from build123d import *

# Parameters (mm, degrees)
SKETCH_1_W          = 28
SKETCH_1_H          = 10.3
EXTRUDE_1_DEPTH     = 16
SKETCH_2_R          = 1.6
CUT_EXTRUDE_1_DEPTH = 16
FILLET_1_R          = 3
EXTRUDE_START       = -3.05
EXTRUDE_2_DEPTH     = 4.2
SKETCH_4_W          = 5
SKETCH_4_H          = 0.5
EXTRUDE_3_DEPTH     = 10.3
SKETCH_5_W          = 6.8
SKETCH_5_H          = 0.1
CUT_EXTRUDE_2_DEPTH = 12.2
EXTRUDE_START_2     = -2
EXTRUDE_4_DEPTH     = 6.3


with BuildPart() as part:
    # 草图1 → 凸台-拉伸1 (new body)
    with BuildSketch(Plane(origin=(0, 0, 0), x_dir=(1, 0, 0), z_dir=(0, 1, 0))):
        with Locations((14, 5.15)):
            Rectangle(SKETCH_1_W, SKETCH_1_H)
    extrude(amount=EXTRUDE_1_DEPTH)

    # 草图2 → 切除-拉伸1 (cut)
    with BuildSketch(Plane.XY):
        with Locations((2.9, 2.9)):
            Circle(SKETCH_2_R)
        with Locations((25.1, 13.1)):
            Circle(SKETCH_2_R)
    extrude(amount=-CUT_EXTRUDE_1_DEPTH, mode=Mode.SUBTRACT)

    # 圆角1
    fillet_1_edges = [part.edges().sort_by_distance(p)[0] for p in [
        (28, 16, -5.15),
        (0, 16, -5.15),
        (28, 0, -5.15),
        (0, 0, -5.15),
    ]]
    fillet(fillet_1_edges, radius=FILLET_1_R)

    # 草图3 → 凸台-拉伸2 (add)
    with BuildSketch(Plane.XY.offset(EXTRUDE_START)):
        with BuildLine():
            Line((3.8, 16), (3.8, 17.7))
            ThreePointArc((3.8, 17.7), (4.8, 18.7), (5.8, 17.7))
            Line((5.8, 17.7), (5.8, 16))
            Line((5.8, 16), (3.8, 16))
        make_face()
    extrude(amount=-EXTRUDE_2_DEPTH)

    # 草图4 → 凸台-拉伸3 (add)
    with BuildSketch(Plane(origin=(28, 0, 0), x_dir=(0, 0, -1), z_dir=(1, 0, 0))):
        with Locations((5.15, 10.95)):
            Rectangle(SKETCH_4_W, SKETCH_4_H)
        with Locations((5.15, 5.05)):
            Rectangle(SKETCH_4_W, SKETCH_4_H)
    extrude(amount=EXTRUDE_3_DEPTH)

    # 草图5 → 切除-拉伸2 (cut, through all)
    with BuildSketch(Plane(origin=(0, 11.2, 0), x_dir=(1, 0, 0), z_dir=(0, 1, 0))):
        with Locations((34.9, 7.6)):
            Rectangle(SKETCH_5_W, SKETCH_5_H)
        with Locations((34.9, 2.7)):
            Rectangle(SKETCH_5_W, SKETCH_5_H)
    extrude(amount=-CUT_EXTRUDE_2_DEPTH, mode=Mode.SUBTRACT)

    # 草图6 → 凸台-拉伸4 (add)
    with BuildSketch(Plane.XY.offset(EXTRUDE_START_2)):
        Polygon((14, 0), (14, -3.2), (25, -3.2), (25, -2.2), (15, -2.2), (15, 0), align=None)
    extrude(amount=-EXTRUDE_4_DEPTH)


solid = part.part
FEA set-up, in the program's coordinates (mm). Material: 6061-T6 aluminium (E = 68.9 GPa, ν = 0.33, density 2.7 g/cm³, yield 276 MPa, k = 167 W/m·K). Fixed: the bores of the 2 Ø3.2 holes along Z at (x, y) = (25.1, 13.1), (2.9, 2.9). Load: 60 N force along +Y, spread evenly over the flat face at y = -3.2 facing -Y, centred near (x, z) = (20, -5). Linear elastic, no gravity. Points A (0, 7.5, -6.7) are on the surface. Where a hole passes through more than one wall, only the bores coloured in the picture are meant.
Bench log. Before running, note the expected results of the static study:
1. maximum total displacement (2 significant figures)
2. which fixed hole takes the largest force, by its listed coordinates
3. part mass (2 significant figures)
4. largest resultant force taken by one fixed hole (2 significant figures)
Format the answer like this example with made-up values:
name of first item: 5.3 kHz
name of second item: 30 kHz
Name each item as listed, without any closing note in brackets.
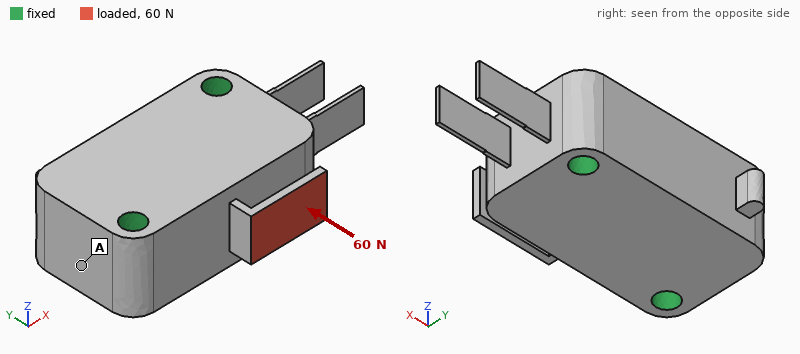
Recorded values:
maximum total displacement: 0.41 mm
which fixed hole takes the largest force, by its listed coordinates: (25.1, 13.1)
part mass: 12 g
largest resultant force taken by one fixed hole: 47 N
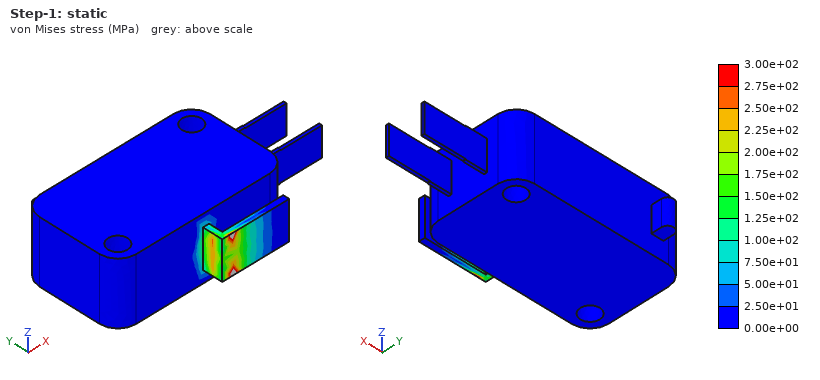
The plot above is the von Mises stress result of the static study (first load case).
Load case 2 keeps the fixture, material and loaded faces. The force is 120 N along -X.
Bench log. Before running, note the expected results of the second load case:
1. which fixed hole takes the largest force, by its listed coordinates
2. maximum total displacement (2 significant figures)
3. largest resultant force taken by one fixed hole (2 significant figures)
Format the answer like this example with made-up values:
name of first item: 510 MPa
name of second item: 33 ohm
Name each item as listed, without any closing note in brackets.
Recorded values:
which fixed hole takes the largest force, by its listed coordinates: (2.9, 2.9)
maximum total displacement: 0.24 mm
largest resultant force taken by one fixed hole: 95 N
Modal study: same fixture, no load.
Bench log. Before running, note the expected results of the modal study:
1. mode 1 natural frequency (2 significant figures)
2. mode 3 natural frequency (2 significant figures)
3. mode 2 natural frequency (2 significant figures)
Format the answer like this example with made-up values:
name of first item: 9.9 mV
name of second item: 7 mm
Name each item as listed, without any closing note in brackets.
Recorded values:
mode 1 natural frequency: 3900 Hz
mode 3 natural frequency: 5500 Hz
mode 2 natural frequency: 3900 Hz
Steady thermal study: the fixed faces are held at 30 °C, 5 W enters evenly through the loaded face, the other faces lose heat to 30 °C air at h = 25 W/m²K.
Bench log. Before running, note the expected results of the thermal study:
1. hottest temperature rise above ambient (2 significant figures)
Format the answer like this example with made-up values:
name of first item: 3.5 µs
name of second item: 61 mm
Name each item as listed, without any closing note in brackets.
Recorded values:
hottest temperature rise above ambient: 39 K
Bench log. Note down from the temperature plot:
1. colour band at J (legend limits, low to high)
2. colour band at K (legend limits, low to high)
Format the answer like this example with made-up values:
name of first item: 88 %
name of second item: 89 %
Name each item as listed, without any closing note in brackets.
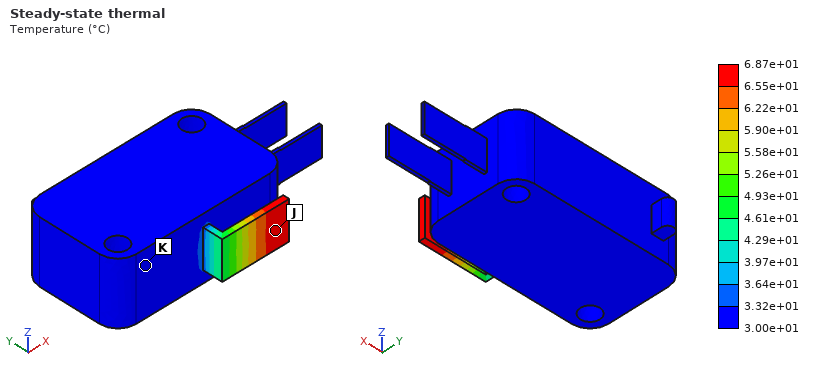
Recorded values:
colour band at J: 6.55e+01 to 6.87e+01 °C
colour band at K: 3.00e+01 to 3.32e+01 °C
